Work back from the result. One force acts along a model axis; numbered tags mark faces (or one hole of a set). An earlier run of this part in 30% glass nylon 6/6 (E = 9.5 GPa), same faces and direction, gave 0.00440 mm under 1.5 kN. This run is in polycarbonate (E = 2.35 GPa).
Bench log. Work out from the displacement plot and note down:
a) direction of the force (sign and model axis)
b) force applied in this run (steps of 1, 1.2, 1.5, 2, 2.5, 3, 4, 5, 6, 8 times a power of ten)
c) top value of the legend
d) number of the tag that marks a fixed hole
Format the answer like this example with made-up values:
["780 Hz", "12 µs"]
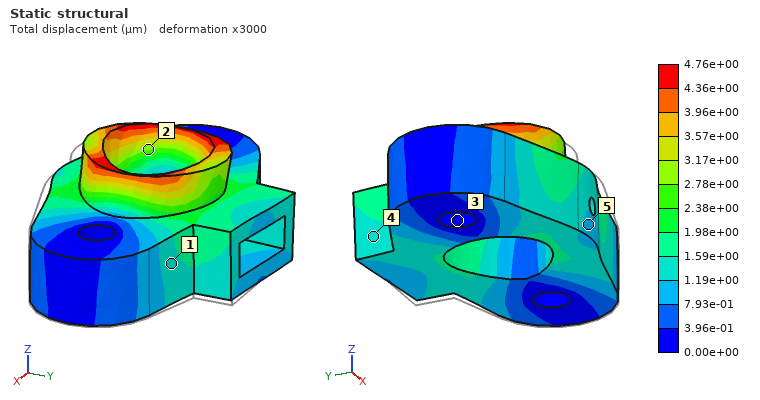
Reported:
["-X", "400 N", "4.76e+00 µm", "3"]
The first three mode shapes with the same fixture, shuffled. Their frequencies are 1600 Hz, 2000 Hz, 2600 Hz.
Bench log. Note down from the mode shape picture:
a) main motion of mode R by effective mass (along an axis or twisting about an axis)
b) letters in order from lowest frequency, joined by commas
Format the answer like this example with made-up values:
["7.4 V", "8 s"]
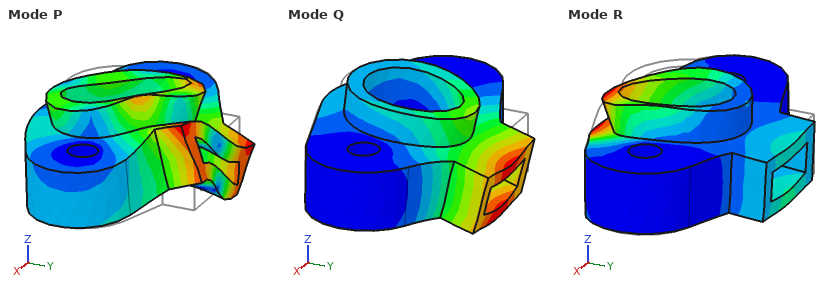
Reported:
["along Z", "Q, R, P"]
